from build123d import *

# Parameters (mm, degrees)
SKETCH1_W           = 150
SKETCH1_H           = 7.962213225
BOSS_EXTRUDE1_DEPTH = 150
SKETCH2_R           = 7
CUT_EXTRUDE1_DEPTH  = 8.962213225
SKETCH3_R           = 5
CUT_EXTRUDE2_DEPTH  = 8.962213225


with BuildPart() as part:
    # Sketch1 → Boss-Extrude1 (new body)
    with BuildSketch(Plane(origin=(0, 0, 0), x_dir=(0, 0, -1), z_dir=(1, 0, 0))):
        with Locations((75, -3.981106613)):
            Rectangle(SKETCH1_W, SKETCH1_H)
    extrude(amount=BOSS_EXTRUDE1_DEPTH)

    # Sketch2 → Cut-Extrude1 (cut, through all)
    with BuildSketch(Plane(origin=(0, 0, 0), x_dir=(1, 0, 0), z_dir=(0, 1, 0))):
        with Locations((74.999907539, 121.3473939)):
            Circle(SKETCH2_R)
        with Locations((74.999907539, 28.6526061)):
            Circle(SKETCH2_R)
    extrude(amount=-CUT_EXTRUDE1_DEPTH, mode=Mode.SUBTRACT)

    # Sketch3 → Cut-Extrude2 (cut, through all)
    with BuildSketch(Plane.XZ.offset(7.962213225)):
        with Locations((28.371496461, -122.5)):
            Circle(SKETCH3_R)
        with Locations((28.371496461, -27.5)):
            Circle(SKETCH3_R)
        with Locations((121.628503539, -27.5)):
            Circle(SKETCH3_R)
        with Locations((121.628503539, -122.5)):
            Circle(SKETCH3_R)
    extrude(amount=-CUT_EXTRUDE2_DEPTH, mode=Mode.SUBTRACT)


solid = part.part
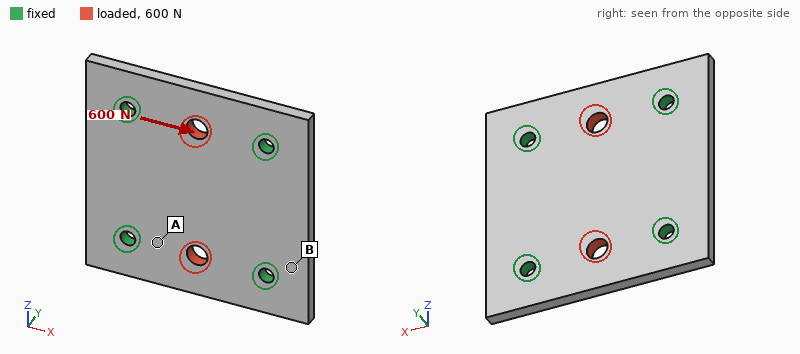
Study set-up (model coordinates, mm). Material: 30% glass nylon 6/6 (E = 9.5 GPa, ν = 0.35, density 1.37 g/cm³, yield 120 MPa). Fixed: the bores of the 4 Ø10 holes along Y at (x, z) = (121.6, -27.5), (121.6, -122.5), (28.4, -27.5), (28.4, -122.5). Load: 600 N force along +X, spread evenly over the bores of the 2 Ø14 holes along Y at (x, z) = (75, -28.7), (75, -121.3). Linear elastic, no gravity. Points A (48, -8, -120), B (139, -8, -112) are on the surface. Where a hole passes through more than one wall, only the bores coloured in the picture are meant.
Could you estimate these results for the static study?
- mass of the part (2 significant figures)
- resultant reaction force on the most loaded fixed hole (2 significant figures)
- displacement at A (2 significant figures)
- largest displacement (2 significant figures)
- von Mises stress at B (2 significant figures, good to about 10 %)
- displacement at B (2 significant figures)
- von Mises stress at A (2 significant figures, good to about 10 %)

240 g
150 N
1.2 µm
2.8 µm
0.17 MPa
0.48 µm
0.64 MPa
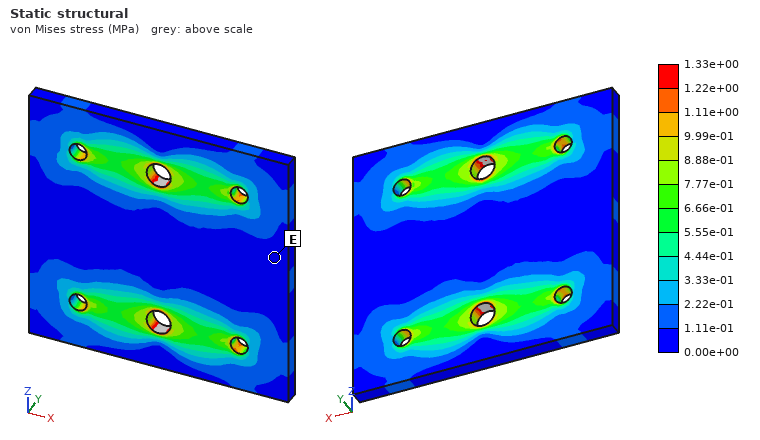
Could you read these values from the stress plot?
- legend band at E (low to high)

0.00e+00 to 1.11e-01 MPa
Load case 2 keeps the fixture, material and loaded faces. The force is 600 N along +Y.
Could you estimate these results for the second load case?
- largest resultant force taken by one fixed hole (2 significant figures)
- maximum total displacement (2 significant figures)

150 N
70 µm
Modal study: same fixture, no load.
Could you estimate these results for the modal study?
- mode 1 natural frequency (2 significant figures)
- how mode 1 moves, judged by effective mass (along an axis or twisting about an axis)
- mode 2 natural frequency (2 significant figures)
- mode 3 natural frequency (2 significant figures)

1800 Hz
along Y
2200 Hz
2200 Hz
